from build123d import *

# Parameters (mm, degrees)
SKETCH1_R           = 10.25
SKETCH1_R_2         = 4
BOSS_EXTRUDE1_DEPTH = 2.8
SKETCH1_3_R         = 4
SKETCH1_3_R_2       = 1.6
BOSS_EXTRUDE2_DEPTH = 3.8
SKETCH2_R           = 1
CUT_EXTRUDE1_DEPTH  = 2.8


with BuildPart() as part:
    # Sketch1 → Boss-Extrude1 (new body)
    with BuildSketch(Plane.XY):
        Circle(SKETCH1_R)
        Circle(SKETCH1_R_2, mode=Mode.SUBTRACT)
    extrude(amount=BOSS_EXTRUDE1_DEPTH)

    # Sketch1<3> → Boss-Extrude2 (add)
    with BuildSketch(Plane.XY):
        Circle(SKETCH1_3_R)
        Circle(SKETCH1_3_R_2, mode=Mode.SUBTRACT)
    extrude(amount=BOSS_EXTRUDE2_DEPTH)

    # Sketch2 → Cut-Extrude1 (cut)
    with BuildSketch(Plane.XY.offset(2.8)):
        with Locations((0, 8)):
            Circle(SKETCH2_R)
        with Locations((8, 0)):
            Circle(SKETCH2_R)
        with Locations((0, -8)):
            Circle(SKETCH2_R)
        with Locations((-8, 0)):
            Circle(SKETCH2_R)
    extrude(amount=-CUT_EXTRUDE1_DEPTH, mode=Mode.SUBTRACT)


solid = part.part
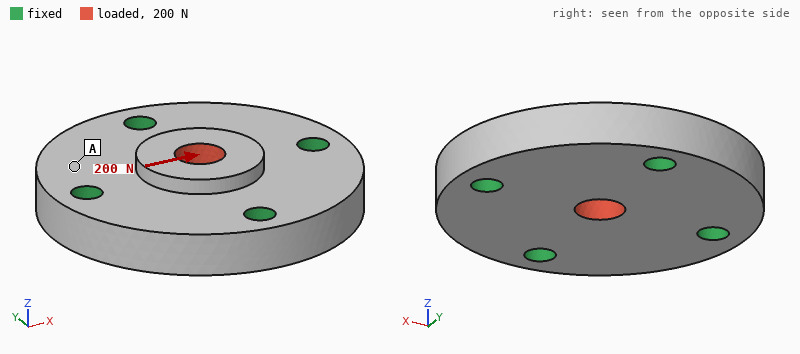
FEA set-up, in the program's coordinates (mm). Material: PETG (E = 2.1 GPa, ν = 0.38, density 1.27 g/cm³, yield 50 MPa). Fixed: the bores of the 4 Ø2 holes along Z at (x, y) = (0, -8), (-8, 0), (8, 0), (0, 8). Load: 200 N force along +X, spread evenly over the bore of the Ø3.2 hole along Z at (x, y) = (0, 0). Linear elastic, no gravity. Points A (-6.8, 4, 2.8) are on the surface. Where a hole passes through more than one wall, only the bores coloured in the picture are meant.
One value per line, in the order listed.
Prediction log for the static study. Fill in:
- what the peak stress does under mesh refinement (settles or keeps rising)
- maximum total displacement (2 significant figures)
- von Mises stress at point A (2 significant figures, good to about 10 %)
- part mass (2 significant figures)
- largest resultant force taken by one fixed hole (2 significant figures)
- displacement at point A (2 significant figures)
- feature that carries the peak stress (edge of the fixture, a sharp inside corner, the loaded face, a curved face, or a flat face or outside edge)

keeps rising
20 µm
1.1 MPa
1.2 g
68 N
6.4 µm
edge of the fixture
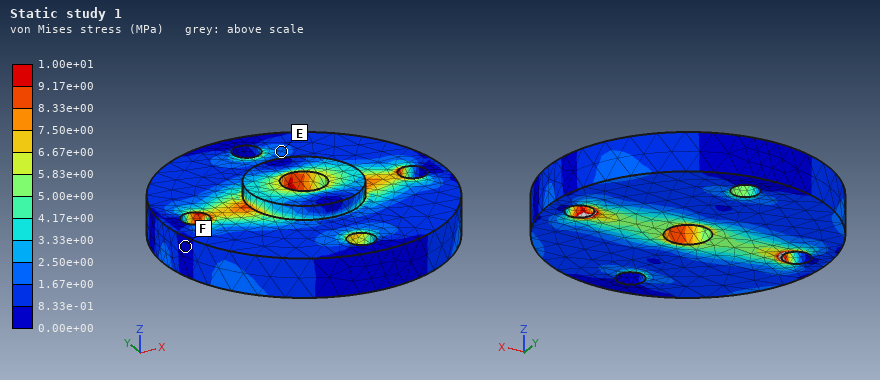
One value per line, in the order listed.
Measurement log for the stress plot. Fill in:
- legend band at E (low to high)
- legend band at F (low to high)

1.67e+00 to 2.50e+00 MPa
0.00e+00 to 8.33e-01 MPa
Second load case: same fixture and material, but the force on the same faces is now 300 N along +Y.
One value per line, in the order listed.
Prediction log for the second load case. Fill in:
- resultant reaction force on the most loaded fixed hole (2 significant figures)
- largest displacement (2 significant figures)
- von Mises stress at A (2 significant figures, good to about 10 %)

100 N
30 µm
1.9 MPa
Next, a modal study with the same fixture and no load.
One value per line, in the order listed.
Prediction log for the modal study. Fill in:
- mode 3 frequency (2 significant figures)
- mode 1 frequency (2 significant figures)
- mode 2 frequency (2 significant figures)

19 kHz
18 kHz
19 kHz
